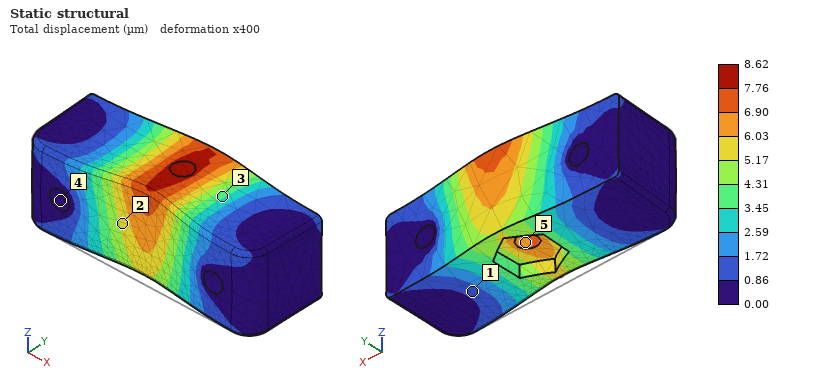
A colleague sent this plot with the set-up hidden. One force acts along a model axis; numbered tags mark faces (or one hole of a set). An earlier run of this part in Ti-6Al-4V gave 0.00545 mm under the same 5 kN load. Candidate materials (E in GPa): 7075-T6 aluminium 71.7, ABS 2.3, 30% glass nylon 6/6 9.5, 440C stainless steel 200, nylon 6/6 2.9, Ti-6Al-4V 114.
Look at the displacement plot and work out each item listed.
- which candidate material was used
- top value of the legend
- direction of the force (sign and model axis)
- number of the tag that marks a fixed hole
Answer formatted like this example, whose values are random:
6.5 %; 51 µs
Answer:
7075-T6 aluminium; 8.62 µm; +Y; 4
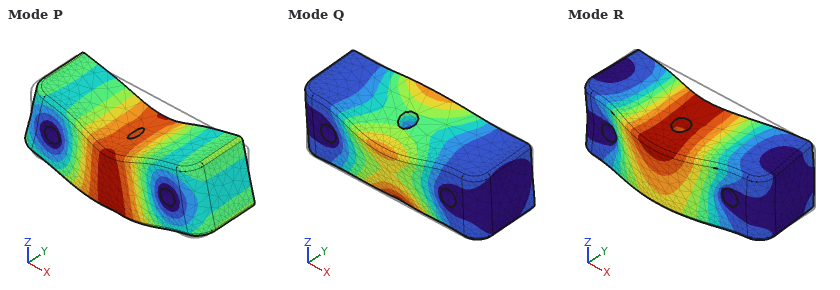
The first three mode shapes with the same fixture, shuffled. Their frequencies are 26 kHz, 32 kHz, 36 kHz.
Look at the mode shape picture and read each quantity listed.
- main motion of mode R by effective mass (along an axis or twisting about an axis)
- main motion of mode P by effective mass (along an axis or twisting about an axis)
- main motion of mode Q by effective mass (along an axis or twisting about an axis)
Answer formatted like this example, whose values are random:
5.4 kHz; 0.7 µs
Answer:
along Y; along Z; twisting about X
